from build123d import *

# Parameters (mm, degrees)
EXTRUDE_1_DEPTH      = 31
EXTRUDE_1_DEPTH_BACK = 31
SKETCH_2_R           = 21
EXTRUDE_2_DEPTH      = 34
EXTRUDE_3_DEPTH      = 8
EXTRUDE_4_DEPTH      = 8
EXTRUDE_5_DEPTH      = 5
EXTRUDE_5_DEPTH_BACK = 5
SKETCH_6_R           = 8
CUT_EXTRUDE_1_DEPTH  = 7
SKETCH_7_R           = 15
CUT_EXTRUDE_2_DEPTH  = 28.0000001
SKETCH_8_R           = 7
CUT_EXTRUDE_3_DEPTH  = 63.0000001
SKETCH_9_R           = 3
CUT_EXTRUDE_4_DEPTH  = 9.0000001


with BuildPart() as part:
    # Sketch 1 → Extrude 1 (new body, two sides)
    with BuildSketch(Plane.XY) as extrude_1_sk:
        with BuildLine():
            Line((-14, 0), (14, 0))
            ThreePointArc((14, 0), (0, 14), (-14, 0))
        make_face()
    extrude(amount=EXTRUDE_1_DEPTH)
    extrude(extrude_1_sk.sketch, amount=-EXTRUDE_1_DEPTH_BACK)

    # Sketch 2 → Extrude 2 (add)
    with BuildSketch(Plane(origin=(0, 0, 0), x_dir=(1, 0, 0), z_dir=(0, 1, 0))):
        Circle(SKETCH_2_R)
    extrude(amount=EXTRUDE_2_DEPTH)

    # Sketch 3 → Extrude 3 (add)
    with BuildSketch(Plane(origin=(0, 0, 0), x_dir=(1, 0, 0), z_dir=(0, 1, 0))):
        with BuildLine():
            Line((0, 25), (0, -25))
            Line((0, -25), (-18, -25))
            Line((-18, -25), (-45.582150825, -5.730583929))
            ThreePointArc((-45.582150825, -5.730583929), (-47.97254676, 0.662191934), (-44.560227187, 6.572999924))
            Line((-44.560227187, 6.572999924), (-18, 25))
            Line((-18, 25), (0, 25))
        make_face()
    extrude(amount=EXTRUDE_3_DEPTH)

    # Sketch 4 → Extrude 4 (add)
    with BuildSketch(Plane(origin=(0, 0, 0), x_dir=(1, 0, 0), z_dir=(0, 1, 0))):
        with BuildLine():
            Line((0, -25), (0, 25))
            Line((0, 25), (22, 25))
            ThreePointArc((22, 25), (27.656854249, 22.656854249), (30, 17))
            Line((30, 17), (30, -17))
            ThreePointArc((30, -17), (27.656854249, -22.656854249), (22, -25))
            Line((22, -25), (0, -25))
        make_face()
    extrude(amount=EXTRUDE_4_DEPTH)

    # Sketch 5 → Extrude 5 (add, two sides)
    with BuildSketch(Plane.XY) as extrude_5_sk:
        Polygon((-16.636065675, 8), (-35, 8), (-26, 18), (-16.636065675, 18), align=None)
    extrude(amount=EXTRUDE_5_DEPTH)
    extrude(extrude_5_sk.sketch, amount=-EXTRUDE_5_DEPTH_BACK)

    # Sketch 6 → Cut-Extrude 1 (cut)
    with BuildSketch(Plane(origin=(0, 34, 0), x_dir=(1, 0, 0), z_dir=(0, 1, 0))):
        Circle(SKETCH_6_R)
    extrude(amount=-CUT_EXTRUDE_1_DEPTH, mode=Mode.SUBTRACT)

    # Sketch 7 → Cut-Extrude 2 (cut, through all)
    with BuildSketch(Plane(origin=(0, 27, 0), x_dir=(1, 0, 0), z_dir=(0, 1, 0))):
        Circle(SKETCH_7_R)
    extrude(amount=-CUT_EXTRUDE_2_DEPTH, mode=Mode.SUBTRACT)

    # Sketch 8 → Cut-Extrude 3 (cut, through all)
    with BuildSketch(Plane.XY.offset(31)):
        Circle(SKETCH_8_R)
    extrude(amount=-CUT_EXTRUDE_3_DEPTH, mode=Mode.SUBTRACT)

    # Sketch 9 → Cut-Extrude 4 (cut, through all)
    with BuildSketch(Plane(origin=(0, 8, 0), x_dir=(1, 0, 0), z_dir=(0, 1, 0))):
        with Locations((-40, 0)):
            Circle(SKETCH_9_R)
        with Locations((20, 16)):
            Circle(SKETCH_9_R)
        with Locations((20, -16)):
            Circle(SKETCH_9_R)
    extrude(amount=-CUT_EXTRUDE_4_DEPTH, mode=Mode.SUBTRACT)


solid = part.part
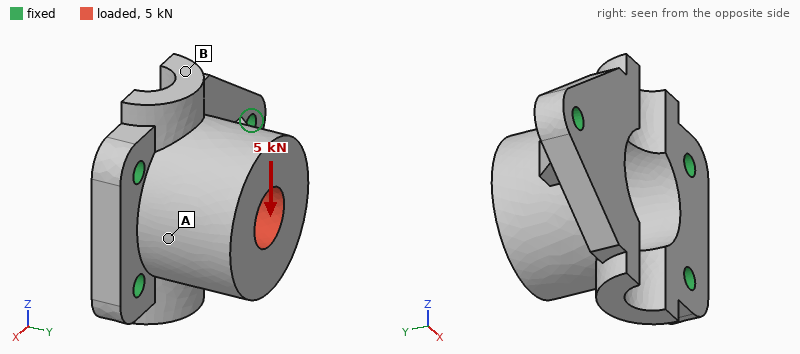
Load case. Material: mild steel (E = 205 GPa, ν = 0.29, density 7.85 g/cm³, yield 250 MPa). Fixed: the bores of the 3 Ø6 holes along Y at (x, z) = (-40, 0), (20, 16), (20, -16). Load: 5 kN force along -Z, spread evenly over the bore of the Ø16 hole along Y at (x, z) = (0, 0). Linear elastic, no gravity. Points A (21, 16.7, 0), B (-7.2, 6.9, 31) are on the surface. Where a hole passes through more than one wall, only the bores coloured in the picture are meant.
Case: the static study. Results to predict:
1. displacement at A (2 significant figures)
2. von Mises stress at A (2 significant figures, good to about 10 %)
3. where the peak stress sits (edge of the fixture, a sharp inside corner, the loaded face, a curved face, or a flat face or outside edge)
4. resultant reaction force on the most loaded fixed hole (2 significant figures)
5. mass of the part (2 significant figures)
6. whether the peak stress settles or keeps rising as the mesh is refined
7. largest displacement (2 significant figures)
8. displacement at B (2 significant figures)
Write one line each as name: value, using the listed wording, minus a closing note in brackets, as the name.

displacement at A: 6.2 µm
von Mises stress at A: 28 MPa
where the peak stress sits: edge of the fixture
resultant reaction force on the most loaded fixed hole: 4.4 kN
mass of the part: 340 g
whether the peak stress settles or keeps rising as the mesh is refined: keeps rising
largest displacement: 20 µm
displacement at B: 13 µm
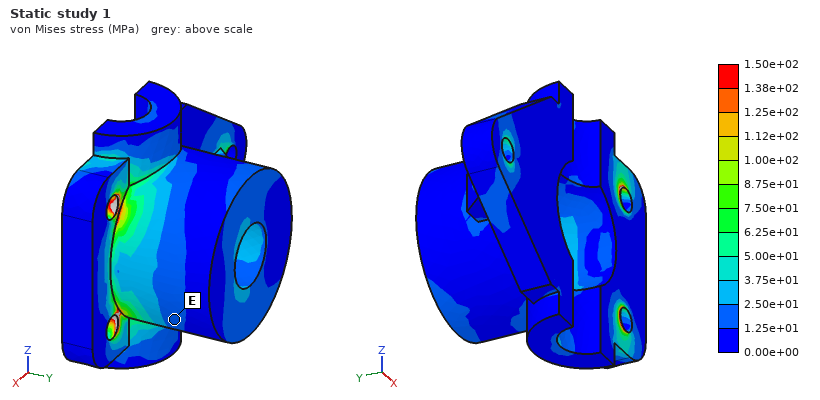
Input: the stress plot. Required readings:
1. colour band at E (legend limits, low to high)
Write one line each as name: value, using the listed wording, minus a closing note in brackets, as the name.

colour band at E: 1.25e+01 to 2.50e+01 MPa
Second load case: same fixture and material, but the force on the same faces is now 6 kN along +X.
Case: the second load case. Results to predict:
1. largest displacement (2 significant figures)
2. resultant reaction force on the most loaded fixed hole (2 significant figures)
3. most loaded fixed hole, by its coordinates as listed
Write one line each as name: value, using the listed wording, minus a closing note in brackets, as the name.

largest displacement: 15 µm
resultant reaction force on the most loaded fixed hole: 4.2 kN
most loaded fixed hole, by its coordinates as listed: (-40, 0)
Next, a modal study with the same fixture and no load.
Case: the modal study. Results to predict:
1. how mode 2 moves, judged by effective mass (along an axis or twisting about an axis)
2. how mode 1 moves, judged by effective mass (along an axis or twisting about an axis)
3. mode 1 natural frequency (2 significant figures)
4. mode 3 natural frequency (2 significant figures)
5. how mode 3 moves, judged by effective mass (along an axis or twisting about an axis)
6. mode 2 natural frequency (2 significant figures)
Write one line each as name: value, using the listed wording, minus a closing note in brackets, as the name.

how mode 2 moves, judged by effective mass: along Y
how mode 1 moves, judged by effective mass: along Z
mode 1 natural frequency: 7500 Hz
mode 3 natural frequency: 12 kHz
how mode 3 moves, judged by effective mass: along Z
mode 2 natural frequency: 8600 Hz
